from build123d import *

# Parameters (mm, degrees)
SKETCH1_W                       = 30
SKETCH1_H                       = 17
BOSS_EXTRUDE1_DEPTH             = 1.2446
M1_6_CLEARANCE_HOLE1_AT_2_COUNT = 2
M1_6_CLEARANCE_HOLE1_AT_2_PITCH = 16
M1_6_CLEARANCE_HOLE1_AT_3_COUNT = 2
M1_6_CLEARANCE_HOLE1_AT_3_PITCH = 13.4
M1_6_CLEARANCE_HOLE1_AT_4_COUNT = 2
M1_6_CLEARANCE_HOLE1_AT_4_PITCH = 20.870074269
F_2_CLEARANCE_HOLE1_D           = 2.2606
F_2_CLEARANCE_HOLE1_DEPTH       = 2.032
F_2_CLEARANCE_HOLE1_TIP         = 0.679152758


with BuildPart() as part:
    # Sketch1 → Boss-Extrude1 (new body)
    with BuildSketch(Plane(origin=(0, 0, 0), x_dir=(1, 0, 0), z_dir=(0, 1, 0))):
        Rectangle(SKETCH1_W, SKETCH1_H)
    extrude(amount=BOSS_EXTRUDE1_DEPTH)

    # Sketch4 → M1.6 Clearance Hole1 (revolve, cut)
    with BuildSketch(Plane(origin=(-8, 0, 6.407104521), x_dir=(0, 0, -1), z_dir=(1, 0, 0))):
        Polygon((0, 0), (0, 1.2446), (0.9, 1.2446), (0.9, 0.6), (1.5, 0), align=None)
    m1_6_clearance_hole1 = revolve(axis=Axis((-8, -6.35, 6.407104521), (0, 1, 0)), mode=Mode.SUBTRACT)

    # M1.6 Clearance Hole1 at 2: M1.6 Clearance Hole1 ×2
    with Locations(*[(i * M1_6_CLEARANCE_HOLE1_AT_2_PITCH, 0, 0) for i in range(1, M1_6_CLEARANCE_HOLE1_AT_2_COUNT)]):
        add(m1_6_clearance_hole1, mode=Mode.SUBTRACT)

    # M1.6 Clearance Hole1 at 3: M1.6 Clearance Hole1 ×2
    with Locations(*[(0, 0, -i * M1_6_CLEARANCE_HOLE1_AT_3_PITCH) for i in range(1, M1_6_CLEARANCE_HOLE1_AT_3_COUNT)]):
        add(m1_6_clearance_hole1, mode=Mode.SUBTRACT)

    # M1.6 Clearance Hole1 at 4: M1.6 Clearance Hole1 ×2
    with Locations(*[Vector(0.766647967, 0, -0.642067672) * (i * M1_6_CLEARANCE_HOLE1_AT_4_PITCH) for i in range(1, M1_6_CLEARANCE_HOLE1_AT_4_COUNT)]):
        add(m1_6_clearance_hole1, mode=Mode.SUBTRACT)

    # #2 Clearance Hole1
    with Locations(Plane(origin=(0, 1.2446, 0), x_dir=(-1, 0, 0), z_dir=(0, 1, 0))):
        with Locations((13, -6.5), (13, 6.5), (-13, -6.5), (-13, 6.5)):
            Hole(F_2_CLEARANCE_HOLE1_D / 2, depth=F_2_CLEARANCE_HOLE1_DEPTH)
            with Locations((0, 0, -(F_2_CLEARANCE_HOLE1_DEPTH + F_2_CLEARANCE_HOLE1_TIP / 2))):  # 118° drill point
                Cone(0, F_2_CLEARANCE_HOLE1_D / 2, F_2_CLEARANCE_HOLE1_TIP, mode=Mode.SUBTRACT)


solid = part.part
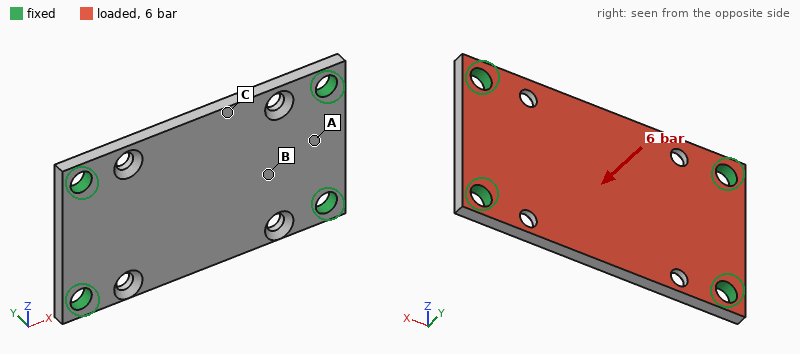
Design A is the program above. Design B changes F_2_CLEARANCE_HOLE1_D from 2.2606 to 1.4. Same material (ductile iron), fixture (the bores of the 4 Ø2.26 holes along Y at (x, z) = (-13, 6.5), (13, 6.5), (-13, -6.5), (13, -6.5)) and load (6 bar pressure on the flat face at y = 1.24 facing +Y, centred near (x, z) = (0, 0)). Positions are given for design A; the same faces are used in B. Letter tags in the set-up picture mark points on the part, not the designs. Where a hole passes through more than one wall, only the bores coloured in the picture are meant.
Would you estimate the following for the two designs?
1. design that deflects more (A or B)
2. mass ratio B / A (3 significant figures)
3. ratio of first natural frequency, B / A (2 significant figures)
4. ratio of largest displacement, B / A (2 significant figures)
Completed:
B
1.02
0.91
1.2
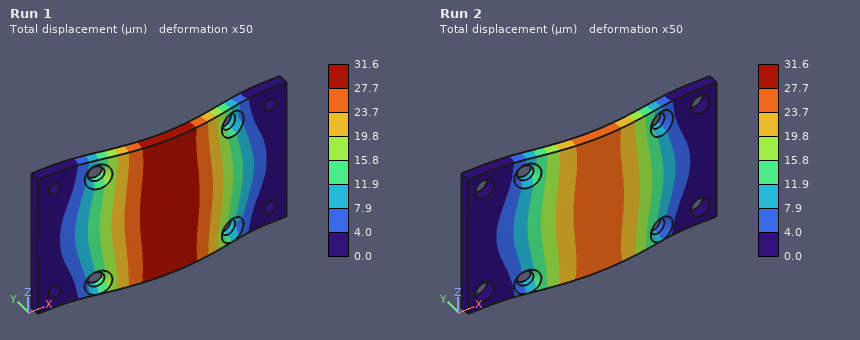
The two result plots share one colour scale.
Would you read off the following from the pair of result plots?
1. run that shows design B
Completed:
Run 1
